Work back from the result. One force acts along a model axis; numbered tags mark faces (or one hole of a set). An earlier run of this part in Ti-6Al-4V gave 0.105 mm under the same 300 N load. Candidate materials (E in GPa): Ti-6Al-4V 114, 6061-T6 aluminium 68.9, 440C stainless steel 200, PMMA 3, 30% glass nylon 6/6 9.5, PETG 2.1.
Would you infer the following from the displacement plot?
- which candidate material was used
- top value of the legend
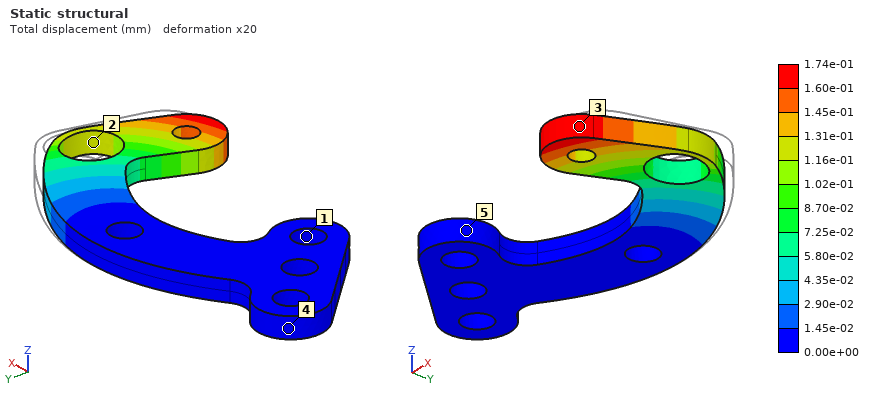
6061-T6 aluminium
1.74e-01 mm
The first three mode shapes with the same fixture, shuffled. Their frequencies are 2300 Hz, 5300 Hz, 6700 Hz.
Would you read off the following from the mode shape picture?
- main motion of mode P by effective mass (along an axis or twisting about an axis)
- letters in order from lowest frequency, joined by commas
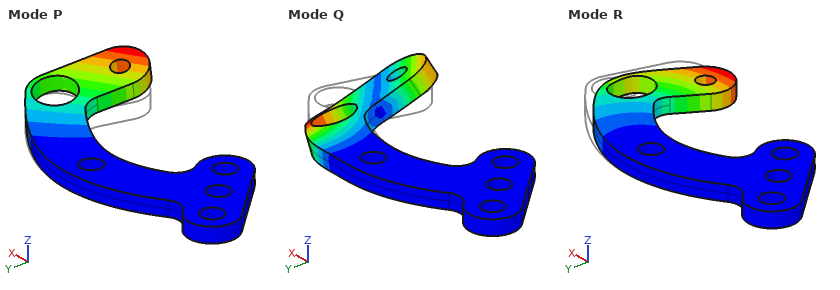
along Z
P, R, Q
